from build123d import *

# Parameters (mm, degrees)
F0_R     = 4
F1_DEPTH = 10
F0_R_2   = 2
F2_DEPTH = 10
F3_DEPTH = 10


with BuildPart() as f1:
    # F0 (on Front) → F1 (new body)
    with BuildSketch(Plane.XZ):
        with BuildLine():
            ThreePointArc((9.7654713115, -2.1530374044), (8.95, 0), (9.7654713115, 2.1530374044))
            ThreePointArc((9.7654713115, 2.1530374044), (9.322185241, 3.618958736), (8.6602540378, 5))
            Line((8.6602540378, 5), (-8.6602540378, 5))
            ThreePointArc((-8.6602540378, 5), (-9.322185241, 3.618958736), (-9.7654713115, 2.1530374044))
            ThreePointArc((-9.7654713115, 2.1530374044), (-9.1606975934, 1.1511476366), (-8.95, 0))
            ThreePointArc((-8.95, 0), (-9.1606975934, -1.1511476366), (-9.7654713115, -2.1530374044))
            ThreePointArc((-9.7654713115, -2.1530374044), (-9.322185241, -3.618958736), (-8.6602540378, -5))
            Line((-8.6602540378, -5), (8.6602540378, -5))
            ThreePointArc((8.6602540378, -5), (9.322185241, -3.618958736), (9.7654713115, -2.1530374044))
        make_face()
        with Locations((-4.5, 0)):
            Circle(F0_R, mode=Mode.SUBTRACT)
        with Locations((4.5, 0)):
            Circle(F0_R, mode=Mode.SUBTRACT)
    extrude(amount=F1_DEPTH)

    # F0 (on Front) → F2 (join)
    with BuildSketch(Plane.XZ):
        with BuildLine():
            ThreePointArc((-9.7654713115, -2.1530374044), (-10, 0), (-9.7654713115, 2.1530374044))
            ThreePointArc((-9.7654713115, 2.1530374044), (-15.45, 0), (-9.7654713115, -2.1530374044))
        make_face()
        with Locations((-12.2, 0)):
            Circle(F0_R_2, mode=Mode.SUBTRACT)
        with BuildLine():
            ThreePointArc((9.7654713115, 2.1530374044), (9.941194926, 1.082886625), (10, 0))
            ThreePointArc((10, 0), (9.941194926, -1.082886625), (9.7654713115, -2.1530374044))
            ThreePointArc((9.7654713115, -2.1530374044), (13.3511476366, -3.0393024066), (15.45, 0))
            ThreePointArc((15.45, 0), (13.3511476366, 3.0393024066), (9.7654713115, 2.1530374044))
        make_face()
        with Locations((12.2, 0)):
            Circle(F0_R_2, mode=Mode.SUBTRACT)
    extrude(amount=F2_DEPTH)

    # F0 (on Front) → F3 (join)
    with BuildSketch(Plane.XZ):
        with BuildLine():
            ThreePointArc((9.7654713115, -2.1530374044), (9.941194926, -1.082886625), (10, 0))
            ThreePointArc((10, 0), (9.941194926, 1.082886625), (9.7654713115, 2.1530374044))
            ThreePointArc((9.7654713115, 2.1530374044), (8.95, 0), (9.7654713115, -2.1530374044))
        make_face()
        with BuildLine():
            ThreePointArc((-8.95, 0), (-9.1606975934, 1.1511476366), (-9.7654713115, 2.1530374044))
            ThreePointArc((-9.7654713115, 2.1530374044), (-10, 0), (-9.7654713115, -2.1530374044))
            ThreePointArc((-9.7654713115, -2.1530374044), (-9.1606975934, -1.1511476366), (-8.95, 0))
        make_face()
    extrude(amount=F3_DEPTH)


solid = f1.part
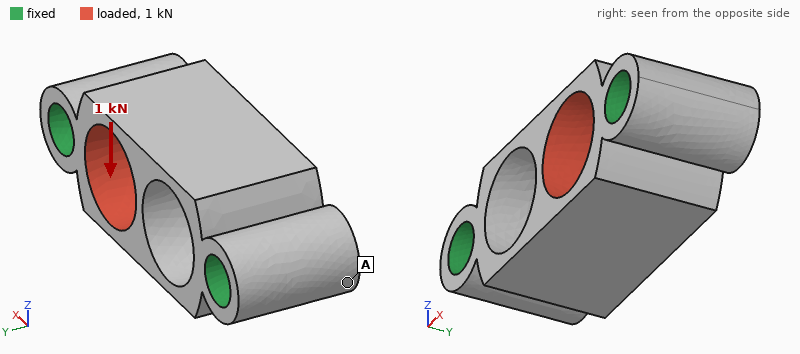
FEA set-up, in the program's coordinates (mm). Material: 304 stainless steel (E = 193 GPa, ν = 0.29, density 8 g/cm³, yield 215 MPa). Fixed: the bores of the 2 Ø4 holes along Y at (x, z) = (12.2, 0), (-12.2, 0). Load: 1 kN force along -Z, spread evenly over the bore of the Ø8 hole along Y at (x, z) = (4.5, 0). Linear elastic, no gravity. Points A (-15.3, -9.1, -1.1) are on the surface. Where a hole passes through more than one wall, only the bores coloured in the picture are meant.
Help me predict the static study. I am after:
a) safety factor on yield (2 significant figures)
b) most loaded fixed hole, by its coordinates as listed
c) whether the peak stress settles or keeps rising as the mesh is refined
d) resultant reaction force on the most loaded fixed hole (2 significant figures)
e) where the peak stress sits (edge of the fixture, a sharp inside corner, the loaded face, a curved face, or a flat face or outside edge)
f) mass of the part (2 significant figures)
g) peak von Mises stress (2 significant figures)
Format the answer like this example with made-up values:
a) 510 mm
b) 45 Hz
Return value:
a) 2.2
b) (12.2, 0)
c) settles
d) 740 N
e) a flat face or outside edge
f) 10 g
g) 99 MPa
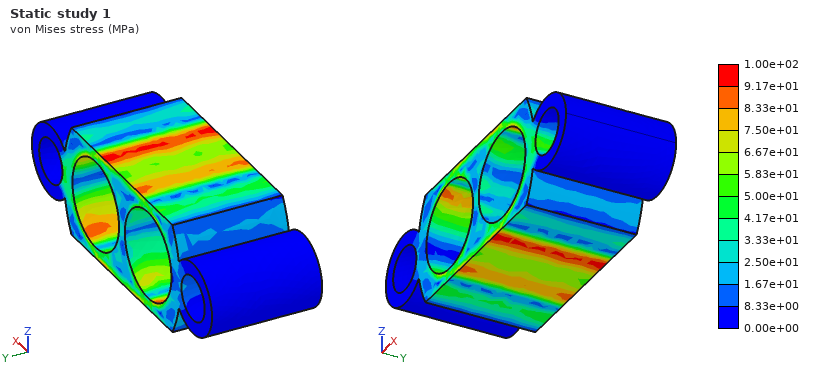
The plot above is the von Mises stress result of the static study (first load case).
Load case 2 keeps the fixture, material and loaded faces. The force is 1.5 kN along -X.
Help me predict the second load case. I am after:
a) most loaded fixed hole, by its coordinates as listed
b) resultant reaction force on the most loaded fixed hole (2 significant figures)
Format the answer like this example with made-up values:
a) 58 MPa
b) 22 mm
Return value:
a) (12.2, 0)
b) 1.0 kN
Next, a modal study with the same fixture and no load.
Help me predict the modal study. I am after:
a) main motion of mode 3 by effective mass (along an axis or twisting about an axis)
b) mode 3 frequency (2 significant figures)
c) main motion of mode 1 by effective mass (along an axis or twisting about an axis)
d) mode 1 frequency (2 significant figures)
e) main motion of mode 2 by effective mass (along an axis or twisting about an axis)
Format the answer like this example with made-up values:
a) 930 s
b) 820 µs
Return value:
a) along Y
b) 44 kHz
c) along Z
d) 24 kHz
e) along X
